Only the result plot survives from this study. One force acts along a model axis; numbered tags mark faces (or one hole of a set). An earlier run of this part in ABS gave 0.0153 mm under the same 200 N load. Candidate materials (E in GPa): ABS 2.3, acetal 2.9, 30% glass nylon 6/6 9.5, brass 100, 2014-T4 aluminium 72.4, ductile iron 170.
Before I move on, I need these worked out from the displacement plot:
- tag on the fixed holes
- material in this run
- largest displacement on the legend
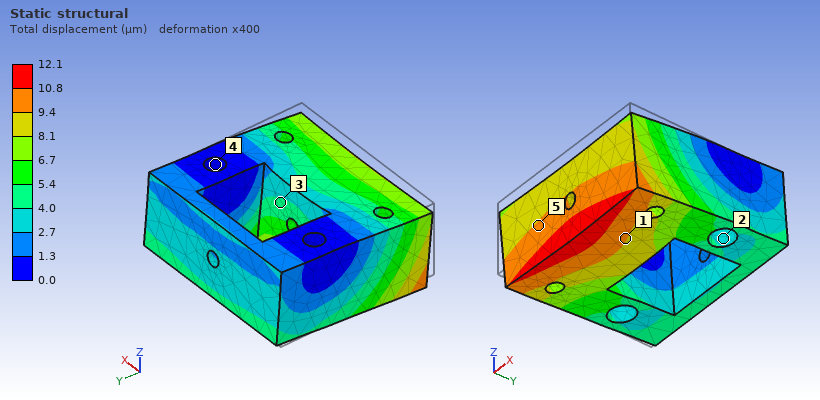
4
acetal
12.1 µm
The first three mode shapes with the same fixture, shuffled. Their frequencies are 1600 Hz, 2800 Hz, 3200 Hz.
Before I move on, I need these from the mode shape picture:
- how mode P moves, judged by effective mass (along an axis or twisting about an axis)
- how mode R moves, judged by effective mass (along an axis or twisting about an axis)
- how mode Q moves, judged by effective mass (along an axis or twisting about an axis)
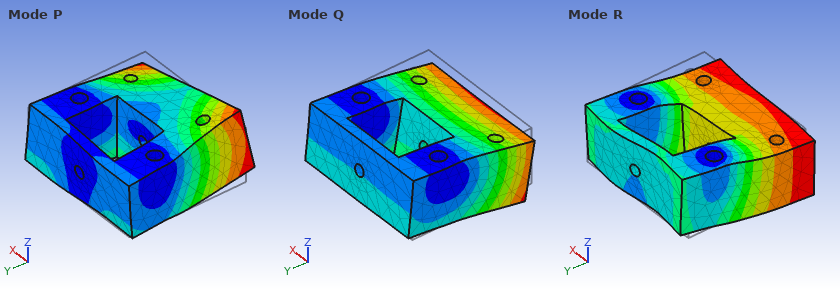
twisting about Y
along X
along Z
